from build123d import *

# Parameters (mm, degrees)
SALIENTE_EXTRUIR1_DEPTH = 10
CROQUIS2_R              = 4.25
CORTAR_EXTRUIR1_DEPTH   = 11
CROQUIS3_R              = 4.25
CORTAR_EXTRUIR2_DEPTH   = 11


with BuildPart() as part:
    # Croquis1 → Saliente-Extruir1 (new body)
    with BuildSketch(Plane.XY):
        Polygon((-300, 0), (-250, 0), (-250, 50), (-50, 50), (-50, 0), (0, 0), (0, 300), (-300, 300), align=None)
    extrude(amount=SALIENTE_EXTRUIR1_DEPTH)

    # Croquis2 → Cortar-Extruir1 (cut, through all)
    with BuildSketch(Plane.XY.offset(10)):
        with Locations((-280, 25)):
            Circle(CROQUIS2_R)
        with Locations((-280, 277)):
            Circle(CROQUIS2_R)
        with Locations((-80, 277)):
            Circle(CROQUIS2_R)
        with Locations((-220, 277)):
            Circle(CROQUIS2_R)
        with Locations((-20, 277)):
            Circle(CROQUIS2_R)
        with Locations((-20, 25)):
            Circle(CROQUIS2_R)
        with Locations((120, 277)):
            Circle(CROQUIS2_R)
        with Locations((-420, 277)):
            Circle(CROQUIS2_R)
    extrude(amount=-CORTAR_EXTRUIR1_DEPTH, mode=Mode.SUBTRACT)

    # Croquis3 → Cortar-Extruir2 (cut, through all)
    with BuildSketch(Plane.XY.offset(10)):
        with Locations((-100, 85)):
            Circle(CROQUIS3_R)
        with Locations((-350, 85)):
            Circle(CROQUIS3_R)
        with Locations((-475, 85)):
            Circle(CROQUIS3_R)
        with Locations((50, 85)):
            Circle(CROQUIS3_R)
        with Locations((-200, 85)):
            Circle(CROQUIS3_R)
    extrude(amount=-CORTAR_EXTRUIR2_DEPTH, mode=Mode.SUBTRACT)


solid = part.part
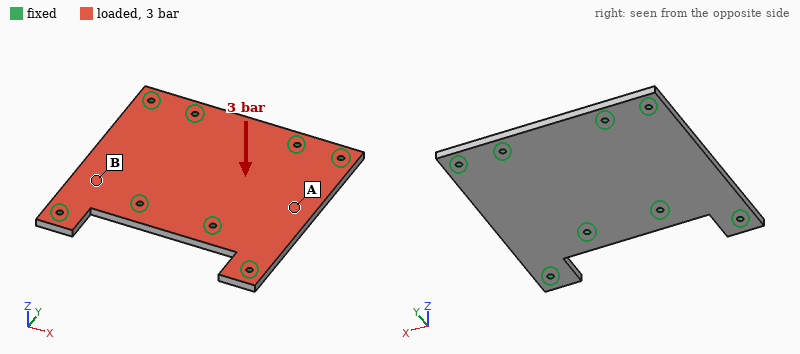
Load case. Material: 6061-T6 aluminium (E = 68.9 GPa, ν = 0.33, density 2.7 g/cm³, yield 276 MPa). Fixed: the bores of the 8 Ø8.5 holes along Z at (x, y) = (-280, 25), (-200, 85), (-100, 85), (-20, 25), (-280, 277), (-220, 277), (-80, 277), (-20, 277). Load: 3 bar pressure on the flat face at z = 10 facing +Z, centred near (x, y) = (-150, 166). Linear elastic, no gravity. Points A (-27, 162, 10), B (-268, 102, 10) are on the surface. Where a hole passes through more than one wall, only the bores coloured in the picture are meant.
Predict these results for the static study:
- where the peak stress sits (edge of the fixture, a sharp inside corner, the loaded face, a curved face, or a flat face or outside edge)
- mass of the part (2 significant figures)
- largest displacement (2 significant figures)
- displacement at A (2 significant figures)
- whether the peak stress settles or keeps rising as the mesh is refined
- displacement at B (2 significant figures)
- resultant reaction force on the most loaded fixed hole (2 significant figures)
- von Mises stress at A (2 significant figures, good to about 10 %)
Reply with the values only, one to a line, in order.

edge of the fixture
2.1 kg
0.44 mm
0.37 mm
keeps rising
0.23 mm
4.7 kN
34 MPa
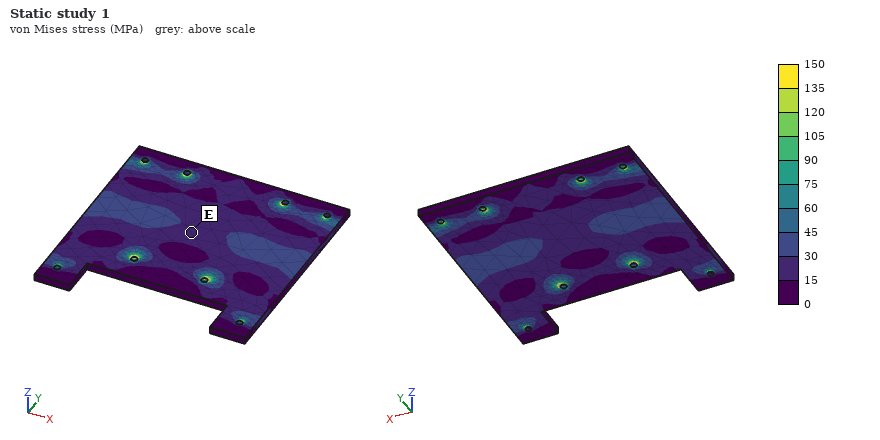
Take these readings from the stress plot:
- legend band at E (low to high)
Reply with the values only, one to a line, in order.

15 to 30 MPa
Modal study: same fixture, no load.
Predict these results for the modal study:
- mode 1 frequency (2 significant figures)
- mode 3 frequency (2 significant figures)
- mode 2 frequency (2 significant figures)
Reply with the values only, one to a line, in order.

1000 Hz
1400 Hz
1100 Hz
